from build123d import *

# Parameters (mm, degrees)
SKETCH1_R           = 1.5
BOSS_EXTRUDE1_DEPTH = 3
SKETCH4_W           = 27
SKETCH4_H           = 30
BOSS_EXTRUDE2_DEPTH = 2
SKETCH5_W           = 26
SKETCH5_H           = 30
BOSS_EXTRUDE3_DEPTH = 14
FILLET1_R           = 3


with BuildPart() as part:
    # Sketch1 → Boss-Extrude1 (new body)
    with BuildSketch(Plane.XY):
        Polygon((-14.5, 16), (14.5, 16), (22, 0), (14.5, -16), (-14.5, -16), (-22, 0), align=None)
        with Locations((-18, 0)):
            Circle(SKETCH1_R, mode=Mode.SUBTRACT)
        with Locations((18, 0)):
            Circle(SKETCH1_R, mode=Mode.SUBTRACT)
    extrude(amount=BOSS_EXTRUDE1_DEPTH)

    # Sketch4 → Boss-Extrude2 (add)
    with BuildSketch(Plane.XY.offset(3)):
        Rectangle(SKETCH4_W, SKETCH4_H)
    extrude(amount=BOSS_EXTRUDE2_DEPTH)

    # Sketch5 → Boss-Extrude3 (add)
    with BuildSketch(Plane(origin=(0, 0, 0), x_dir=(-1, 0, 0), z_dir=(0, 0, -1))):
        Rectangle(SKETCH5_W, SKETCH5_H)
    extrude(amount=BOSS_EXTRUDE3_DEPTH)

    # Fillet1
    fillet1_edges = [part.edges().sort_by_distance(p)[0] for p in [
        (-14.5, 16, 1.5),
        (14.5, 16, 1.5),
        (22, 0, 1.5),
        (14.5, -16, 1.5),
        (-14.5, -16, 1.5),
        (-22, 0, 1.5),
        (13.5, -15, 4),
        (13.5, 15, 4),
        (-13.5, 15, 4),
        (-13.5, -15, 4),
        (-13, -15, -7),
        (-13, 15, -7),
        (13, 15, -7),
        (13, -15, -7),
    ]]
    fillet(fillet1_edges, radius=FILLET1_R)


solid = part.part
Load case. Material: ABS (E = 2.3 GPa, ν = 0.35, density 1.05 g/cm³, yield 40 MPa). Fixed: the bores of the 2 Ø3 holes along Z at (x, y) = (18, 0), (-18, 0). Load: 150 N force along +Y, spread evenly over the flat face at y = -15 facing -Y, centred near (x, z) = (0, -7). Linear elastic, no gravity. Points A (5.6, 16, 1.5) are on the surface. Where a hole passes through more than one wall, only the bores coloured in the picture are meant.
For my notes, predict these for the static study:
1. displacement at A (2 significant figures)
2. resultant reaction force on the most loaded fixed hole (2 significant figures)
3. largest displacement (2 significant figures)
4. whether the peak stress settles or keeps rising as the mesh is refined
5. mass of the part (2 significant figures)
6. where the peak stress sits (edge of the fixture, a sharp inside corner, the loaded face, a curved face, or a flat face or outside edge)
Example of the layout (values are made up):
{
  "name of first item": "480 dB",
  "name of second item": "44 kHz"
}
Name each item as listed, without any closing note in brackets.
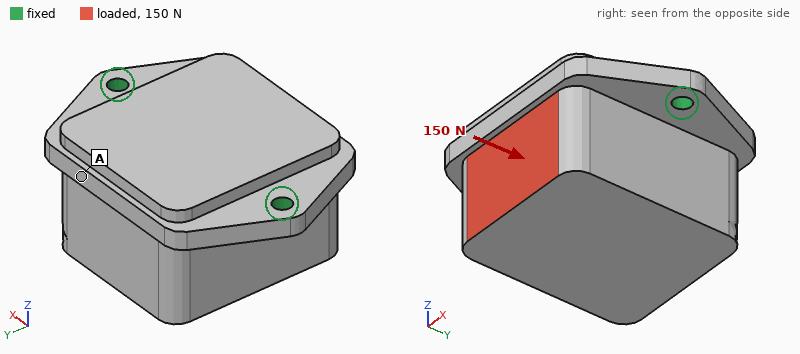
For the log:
{
  "displacement at A": "0.36 mm",
  "resultant reaction force on the most loaded fixed hole": "75 N",
  "largest displacement": "0.50 mm",
  "whether the peak stress settles or keeps rising as the mesh is refined": "keeps rising",
  "mass of the part": "17 g",
  "where the peak stress sits": "edge of the fixture"
}
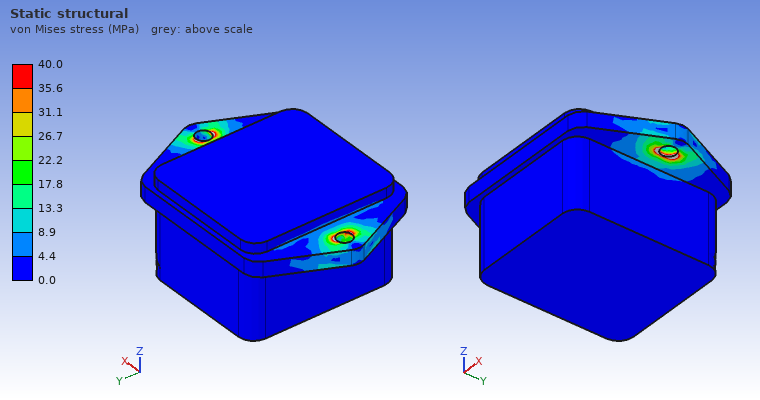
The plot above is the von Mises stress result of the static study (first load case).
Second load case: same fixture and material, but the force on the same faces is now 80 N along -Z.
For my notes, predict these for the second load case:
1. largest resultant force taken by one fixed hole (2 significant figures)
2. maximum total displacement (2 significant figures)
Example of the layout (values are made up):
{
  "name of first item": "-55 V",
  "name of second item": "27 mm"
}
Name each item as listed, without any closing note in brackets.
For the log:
{
  "largest resultant force taken by one fixed hole": "41 N",
  "maximum total displacement": "0.47 mm"
}
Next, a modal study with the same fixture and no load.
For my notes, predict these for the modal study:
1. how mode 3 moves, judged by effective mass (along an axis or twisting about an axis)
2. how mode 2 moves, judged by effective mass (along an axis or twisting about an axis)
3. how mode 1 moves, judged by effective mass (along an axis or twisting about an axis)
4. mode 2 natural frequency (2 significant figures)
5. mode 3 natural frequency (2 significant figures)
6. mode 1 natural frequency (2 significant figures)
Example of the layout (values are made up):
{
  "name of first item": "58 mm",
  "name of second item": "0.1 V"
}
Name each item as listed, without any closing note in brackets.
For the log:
{
  "how mode 3 moves, judged by effective mass": "along X",
  "how mode 2 moves, judged by effective mass": "along Z",
  "how mode 1 moves, judged by effective mass": "along Y",
  "mode 2 natural frequency": "2600 Hz",
  "mode 3 natural frequency": "3400 Hz",
  "mode 1 natural frequency": "800 Hz"
}
